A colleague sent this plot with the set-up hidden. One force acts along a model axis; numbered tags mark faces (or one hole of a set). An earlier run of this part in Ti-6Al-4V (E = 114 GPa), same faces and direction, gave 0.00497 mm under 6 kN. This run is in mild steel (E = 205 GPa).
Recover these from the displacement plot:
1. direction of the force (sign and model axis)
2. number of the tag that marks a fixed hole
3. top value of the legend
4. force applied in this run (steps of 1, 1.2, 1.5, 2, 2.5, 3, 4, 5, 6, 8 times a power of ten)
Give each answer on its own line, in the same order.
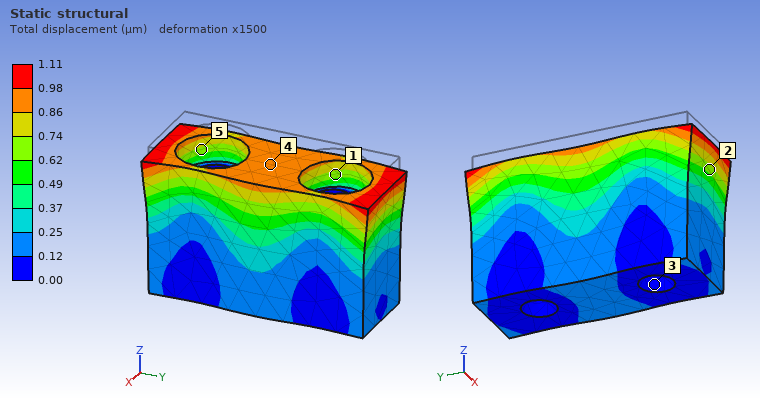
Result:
-Z
3
1.11 µm
2.5 kN
